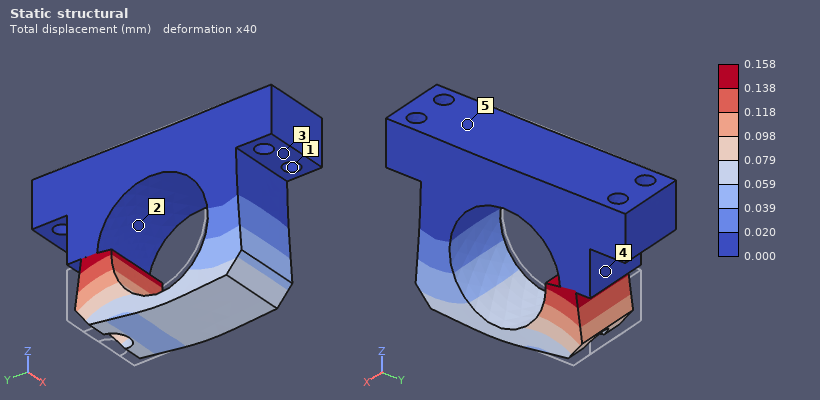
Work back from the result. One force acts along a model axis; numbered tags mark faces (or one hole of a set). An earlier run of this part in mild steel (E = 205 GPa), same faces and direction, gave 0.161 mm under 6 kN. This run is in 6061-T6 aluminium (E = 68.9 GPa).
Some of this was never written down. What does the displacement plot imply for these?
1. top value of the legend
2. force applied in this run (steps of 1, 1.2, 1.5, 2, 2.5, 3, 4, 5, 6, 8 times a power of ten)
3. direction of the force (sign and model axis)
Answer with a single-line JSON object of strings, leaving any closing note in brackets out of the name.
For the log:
{"top value of the legend": "0.158 mm", "force applied in this run": "2 kN", "direction of the force": "-Y"}
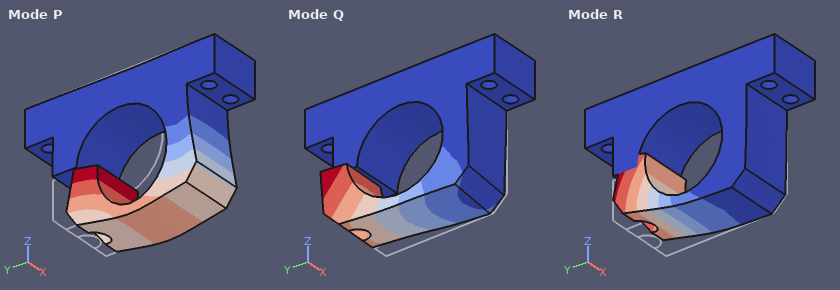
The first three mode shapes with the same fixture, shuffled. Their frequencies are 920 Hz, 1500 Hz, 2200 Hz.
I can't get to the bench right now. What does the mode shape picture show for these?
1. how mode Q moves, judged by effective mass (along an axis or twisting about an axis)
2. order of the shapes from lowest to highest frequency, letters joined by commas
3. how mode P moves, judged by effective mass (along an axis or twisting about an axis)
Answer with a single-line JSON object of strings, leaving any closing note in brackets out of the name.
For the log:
{"how mode Q moves, judged by effective mass": "along X", "order of the shapes from lowest to highest frequency, letters joined by commas": "R, Q, P", "how mode P moves, judged by effective mass": "along Y"}
